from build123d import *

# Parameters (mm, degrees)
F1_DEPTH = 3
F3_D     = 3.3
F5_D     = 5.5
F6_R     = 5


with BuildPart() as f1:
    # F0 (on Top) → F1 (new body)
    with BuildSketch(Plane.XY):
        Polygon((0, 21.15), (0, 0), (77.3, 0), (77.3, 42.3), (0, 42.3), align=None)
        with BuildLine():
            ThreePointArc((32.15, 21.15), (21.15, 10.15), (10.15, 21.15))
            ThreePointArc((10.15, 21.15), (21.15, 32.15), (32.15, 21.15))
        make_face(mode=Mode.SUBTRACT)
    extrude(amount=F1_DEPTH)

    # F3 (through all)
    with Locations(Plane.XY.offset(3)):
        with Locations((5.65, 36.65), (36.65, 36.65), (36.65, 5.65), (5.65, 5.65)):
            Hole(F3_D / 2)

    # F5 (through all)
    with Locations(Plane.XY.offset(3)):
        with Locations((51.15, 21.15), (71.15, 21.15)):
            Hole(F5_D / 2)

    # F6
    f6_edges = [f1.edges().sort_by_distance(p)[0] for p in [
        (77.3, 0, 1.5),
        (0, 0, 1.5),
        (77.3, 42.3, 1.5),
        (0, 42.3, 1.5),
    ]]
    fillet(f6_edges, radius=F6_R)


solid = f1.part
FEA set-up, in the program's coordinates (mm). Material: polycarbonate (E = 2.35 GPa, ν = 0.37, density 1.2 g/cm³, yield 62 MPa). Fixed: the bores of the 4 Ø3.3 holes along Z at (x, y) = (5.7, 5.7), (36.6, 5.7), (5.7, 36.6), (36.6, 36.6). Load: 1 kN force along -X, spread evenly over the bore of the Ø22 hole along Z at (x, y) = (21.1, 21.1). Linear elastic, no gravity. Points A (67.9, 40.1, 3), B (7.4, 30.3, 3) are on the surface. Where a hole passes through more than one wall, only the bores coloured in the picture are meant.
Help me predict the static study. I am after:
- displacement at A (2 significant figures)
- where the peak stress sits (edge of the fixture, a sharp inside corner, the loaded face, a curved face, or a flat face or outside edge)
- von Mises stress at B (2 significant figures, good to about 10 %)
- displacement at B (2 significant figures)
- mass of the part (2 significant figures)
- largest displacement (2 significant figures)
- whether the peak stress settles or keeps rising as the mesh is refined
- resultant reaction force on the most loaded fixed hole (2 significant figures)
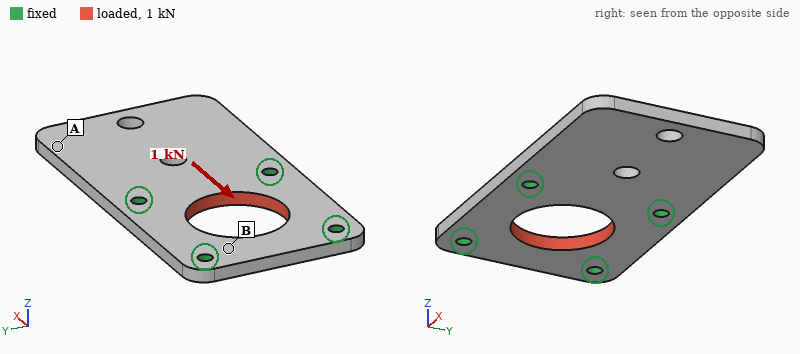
17 µm
edge of the fixture
7.0 MPa
48 µm
10 g
98 µm
keeps rising
260 N
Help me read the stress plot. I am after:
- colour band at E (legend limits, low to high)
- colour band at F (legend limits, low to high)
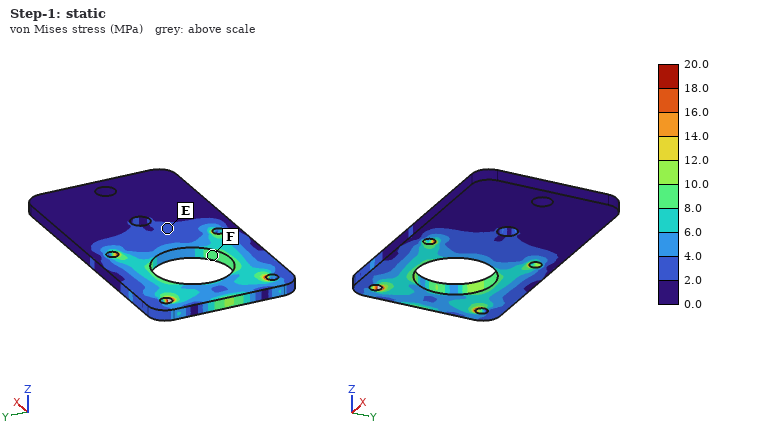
2.0 to 4.0 MPa
8.0 to 10.0 MPa
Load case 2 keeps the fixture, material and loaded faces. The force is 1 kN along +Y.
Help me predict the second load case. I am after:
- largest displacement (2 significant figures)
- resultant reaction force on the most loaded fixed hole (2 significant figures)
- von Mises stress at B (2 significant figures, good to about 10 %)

89 µm
260 N
7.2 MPa
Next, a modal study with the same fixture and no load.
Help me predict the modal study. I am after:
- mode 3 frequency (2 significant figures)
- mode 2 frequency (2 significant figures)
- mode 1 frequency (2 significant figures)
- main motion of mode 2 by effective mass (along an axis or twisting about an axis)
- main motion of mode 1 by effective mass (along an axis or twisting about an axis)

2400 Hz
970 Hz
400 Hz
twisting about X
along Z
